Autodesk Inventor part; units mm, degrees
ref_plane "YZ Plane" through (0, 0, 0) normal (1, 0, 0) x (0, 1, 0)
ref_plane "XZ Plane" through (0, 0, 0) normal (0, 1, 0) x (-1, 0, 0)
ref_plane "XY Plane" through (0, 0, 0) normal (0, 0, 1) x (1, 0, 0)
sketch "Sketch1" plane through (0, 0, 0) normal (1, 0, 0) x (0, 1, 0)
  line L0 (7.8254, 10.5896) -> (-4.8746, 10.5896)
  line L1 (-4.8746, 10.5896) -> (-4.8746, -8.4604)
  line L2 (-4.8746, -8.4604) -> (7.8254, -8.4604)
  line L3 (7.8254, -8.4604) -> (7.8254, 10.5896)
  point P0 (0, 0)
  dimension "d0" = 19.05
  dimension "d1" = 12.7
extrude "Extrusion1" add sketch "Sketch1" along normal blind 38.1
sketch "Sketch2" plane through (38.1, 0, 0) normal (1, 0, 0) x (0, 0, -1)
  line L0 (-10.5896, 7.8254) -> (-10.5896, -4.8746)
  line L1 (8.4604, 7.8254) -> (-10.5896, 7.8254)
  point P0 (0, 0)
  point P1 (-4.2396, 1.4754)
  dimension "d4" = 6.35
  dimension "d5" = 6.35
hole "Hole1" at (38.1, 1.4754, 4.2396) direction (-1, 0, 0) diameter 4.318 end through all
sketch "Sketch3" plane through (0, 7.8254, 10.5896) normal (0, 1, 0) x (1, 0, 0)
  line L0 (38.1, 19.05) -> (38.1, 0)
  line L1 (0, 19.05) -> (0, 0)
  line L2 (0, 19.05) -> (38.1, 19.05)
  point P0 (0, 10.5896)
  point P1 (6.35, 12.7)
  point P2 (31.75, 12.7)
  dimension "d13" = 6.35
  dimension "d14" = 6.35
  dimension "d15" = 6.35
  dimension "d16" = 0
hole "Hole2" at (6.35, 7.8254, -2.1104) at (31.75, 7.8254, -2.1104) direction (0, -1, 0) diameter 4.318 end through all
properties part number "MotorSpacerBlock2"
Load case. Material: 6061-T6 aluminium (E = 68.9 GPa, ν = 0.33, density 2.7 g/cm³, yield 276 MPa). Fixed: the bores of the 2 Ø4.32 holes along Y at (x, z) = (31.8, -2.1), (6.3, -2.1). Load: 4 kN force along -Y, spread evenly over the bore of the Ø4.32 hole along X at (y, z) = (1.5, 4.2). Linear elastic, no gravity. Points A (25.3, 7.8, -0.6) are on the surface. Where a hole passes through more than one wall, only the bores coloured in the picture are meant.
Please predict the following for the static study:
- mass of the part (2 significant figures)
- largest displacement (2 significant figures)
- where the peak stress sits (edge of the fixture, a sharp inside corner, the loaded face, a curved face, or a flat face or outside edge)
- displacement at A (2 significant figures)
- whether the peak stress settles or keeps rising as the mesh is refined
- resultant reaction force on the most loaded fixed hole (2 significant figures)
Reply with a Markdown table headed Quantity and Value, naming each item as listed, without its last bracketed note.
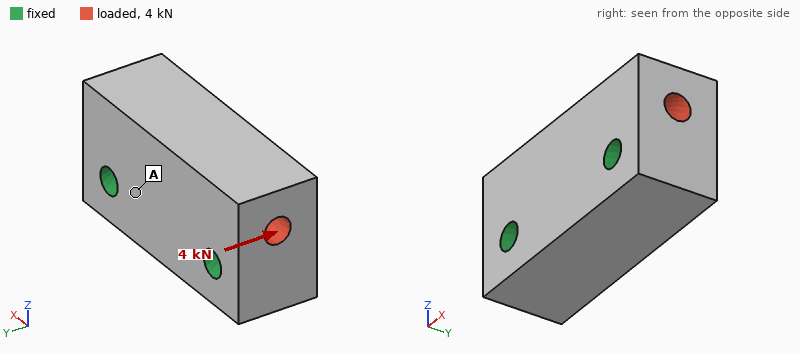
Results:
| Quantity | Value |
|---|---|
| mass of the part | 22 g |
| largest displacement | 9.4 µm |
| where the peak stress sits | edge of the fixture |
| displacement at A | 3.4 µm |
| whether the peak stress settles or keeps rising as the mesh is refined | keeps rising |
| resultant reaction force on the most loaded fixed hole | 2.0 kN |
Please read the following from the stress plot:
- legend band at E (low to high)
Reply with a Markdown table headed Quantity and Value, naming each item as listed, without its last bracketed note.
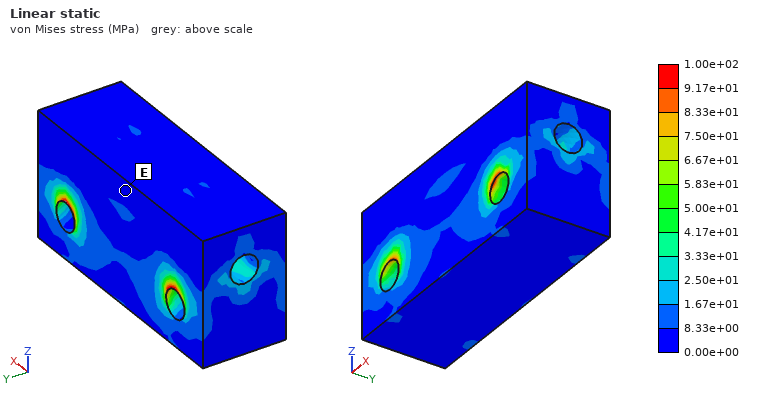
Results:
| Quantity | Value |
|---|---|
| legend band at E | 0.00e+00 to 8.33e+00 MPa |
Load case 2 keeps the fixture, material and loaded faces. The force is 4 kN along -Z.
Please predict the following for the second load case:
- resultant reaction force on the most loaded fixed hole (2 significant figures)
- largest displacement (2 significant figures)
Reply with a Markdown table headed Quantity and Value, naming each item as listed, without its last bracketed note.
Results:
| Quantity | Value |
|---|---|
| resultant reaction force on the most loaded fixed hole | 2.0 kN |
| largest displacement | 3.1 µm |
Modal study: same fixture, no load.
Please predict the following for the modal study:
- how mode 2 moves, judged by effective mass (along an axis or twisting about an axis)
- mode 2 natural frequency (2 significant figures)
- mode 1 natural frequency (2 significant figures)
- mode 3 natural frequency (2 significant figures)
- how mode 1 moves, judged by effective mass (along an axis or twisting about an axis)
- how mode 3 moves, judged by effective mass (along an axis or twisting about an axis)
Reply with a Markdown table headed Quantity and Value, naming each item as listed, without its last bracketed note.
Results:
| Quantity | Value |
|---|---|
| how mode 2 moves, judged by effective mass | twisting about Z |
| mode 2 natural frequency | 44 kHz |
| mode 1 natural frequency | 31 kHz |
| mode 3 natural frequency | 47 kHz |
| how mode 1 moves, judged by effective mass | along Y |
| how mode 3 moves, judged by effective mass | along Z |
